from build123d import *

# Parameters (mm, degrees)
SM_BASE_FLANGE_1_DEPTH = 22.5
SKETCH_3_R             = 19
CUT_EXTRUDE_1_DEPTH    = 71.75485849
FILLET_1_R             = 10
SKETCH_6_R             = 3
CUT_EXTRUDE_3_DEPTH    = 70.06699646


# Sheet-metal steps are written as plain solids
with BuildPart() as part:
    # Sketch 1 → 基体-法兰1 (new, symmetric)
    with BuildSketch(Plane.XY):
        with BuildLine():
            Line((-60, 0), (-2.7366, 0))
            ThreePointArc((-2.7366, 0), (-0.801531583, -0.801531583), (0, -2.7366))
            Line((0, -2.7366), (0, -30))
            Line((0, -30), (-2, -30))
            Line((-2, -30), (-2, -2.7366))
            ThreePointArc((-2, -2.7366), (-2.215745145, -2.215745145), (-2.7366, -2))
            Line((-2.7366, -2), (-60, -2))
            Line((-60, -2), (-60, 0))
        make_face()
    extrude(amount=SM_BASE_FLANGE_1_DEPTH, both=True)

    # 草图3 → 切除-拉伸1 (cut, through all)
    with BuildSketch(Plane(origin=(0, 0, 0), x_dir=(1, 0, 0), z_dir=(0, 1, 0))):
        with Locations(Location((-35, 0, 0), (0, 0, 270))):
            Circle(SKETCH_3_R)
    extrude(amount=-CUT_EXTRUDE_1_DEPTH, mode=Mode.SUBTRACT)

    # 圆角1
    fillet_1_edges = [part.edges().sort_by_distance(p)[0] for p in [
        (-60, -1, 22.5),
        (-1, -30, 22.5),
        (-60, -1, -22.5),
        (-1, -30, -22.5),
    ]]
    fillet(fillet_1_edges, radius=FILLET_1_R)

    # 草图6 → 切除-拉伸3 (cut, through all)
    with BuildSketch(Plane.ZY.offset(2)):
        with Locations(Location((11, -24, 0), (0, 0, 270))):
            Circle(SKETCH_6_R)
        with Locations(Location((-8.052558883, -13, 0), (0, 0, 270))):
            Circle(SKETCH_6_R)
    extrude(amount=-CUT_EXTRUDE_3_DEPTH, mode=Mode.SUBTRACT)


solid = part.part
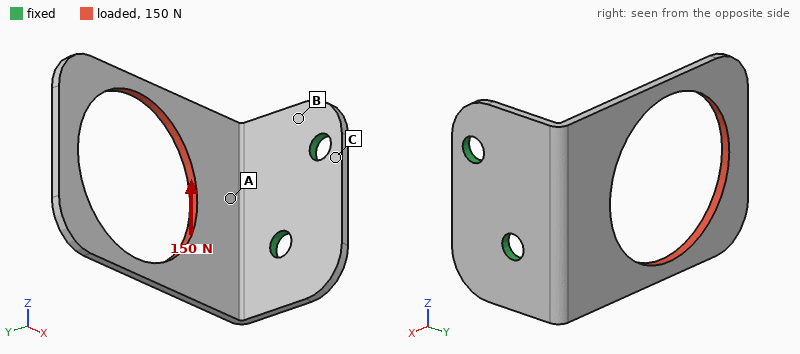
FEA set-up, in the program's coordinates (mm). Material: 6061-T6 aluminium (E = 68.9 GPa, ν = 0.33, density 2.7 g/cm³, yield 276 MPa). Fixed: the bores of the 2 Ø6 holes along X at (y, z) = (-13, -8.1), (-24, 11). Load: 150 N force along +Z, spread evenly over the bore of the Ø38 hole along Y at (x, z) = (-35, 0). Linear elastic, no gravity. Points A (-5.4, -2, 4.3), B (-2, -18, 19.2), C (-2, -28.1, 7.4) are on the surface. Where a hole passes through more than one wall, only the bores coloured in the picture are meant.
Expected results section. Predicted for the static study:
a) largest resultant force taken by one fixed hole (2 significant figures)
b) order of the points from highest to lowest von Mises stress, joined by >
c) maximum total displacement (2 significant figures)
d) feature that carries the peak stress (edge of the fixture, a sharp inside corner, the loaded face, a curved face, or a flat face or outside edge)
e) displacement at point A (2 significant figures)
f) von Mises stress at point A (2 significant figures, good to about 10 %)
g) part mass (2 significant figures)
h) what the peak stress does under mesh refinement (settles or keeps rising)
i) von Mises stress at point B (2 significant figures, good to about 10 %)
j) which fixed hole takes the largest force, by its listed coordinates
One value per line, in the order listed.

190 N
B > A > C
0.83 mm
edge of the fixture
0.13 mm
46 MPa
14 g
keeps rising
80 MPa
(-13, -8.1)
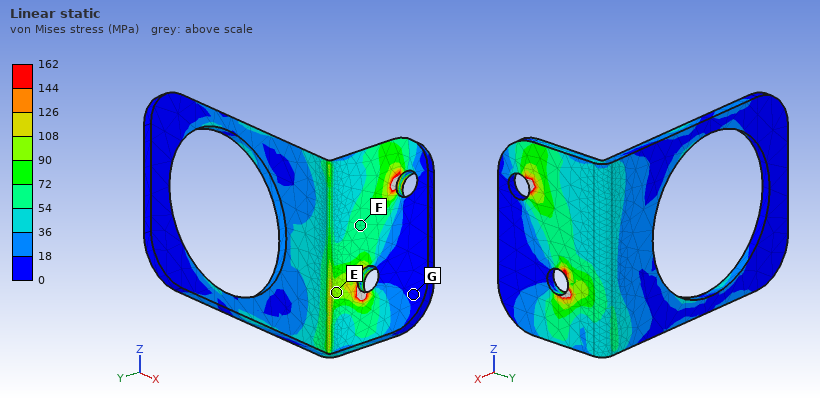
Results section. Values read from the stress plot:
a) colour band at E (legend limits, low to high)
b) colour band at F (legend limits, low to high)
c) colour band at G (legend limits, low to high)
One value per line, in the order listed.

90 to 108 MPa
54 to 72 MPa
0 to 18 MPa
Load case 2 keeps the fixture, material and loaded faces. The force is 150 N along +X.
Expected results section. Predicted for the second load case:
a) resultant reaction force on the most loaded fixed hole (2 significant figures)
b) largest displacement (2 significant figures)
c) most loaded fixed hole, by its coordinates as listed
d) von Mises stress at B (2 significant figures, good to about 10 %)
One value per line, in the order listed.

130 N
0.40 mm
(-13, -8.1)
30 MPa
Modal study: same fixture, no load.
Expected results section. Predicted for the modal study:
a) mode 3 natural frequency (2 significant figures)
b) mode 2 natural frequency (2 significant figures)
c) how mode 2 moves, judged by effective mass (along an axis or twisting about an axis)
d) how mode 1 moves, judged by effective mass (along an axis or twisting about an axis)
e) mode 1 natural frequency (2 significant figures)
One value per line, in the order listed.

1200 Hz
970 Hz
along Z
along Y
390 Hz
